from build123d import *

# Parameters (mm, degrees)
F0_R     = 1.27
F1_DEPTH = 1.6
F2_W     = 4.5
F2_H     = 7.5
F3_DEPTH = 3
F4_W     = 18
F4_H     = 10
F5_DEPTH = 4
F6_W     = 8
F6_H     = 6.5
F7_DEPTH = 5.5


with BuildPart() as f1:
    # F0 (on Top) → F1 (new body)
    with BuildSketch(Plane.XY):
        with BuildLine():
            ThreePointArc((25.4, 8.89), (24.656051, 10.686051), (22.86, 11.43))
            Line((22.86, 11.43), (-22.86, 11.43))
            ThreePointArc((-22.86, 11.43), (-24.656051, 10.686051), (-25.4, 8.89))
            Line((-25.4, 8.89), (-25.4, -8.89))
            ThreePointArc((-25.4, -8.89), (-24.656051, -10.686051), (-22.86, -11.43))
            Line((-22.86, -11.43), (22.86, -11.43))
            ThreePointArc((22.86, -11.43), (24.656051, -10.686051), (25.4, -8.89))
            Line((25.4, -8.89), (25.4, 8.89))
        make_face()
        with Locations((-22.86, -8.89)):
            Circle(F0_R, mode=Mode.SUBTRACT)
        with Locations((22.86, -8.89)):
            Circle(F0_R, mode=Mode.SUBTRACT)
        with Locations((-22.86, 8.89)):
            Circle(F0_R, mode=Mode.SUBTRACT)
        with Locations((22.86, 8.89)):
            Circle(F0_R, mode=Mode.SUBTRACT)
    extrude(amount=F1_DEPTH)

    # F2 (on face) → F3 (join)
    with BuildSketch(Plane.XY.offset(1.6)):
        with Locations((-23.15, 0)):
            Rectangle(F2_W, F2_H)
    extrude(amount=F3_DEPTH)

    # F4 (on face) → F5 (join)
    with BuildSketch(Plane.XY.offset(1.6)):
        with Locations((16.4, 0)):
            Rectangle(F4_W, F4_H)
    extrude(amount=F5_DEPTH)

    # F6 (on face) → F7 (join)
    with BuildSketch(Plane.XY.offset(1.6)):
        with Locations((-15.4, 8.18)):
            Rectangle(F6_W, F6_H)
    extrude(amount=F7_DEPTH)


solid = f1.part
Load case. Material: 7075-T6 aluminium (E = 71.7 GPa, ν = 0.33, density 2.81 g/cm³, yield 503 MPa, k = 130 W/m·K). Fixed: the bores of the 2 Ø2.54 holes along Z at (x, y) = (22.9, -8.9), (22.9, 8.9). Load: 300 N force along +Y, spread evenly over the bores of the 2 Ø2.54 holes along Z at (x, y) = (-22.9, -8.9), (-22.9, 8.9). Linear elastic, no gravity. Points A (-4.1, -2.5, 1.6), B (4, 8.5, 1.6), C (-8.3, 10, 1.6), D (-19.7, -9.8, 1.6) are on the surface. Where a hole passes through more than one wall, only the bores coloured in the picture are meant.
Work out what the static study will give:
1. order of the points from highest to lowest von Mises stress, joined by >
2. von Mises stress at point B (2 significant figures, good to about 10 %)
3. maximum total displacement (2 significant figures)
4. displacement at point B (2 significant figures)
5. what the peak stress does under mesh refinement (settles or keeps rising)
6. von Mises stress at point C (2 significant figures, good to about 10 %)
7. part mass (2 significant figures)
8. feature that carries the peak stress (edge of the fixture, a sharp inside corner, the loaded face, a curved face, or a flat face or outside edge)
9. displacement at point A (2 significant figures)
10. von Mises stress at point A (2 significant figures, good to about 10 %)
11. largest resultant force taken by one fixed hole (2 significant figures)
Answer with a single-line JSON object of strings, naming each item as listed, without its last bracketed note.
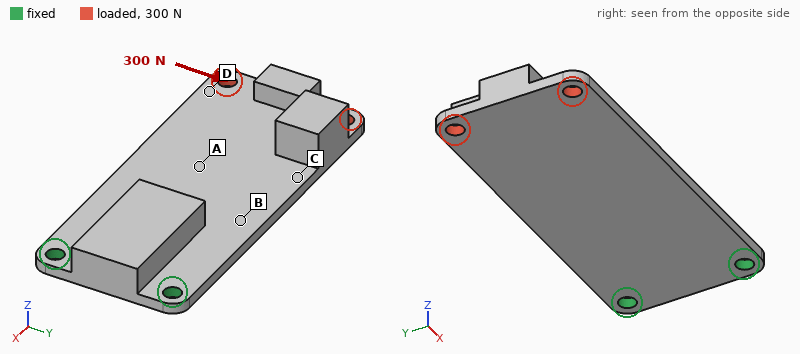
{"order of the points from highest to lowest von Mises stress, joined by >": "B > C > A > D", "von Mises stress at point B": "43 MPa", "maximum total displacement": "0.11 mm", "displacement at point B": "0.027 mm", "what the peak stress does under mesh refinement": "keeps rising", "von Mises stress at point C": "30 MPa", "part mass": "8.2 g", "feature that carries the peak stress": "edge of the fixture", "displacement at point A": "0.041 mm", "von Mises stress at point A": "22 MPa", "largest resultant force taken by one fixed hole": "770 N"}
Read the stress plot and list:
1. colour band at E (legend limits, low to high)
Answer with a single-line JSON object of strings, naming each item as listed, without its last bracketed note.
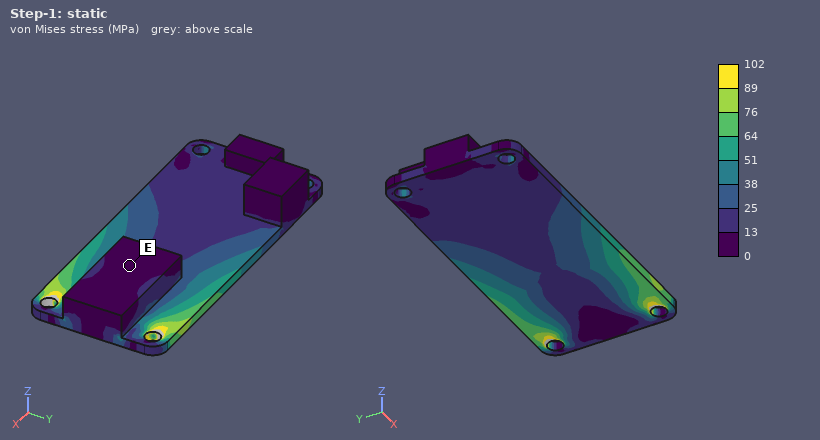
{"colour band at E": "0 to 13 MPa"}
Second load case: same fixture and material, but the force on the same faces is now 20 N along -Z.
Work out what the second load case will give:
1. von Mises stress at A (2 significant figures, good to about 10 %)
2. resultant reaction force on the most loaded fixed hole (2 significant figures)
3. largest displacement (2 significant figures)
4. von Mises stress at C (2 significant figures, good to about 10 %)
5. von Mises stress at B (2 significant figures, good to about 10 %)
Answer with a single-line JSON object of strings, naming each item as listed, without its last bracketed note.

{"von Mises stress at A": "35 MPa", "resultant reaction force on the most loaded fixed hole": "12 N", "largest displacement": "0.62 mm", "von Mises stress at C": "32 MPa", "von Mises stress at B": "47 MPa"}
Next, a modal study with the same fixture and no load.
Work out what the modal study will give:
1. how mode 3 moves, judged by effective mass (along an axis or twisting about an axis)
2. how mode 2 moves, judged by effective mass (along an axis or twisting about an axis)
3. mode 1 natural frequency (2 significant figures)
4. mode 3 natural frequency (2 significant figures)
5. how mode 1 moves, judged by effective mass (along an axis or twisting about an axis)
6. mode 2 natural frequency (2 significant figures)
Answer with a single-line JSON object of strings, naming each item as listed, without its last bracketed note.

{"how mode 3 moves, judged by effective mass": "along Z", "how mode 2 moves, judged by effective mass": "twisting about X", "mode 1 natural frequency": "670 Hz", "mode 3 natural frequency": "3400 Hz", "how mode 1 moves, judged by effective mass": "along Z", "mode 2 natural frequency": "2800 Hz"}
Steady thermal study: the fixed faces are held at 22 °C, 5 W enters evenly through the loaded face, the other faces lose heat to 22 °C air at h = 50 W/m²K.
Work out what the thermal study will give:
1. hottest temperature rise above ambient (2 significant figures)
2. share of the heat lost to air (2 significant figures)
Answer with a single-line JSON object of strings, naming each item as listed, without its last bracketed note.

{"hottest temperature rise above ambient": "36 K", "share of the heat lost to air": "42 %"}
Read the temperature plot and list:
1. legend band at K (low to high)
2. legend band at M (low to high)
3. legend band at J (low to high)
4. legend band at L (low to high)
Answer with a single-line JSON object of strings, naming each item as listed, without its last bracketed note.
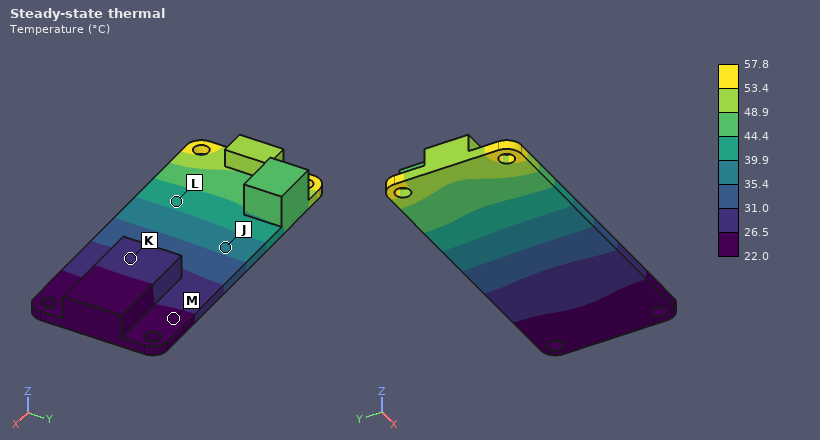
{"legend band at K": "26.5 to 31.0 °C", "legend band at M": "22.0 to 26.5 °C", "legend band at J": "35.4 to 39.9 °C", "legend band at L": "39.9 to 44.4 °C"}
